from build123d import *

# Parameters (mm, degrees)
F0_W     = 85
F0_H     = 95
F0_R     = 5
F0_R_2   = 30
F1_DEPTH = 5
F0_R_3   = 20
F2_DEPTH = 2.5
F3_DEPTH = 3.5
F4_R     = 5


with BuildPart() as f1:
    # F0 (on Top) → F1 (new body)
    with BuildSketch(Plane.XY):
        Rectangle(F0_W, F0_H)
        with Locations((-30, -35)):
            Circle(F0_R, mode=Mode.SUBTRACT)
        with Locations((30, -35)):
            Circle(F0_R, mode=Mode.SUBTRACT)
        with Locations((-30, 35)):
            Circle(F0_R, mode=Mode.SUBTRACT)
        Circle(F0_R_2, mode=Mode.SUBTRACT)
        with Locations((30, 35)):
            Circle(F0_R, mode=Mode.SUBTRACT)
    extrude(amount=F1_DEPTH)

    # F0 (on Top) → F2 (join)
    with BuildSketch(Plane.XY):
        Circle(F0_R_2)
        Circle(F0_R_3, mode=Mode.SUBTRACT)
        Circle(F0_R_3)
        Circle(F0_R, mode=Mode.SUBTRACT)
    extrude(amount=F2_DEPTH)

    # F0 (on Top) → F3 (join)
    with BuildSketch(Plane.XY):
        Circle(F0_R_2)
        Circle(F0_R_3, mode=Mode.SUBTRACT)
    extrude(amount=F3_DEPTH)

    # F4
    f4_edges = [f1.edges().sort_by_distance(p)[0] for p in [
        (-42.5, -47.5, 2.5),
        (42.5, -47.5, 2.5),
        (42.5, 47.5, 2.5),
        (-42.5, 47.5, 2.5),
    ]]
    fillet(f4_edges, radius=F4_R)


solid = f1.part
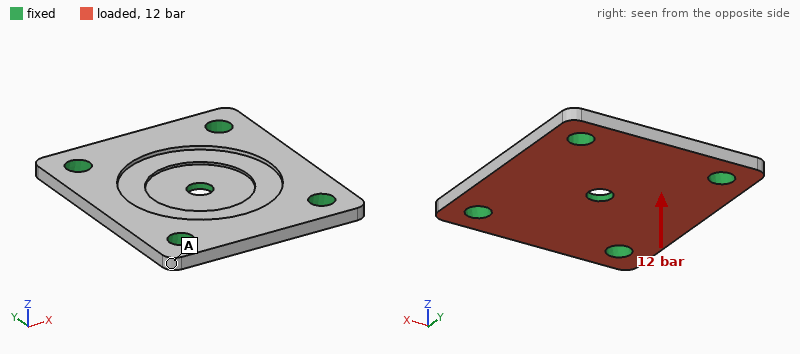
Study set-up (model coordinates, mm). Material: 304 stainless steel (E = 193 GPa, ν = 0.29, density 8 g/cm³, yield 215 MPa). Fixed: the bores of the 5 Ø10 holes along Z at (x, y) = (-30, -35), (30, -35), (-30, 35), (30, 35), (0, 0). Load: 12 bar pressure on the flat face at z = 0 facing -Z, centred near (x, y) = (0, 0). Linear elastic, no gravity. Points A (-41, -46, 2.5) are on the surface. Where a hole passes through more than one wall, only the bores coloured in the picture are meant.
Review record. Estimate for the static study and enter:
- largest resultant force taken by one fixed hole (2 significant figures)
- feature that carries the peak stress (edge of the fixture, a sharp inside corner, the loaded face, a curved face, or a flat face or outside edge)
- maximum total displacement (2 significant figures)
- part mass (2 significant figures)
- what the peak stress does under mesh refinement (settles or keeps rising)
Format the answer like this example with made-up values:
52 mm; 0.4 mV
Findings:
1.9 kN; edge of the fixture; 28 µm; 260 g; keeps rising
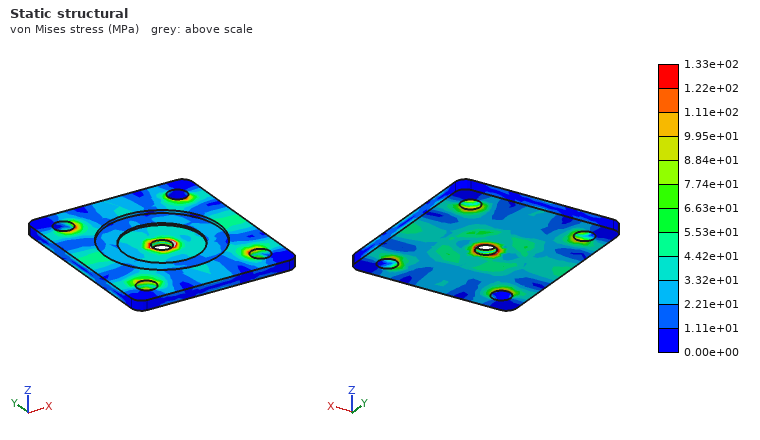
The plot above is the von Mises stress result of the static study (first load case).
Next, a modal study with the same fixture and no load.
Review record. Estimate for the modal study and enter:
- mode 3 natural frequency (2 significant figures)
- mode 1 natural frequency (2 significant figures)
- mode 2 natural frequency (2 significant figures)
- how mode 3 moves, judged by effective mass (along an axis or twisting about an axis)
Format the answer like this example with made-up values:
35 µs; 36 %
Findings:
8600 Hz; 6600 Hz; 6600 Hz; along Z
